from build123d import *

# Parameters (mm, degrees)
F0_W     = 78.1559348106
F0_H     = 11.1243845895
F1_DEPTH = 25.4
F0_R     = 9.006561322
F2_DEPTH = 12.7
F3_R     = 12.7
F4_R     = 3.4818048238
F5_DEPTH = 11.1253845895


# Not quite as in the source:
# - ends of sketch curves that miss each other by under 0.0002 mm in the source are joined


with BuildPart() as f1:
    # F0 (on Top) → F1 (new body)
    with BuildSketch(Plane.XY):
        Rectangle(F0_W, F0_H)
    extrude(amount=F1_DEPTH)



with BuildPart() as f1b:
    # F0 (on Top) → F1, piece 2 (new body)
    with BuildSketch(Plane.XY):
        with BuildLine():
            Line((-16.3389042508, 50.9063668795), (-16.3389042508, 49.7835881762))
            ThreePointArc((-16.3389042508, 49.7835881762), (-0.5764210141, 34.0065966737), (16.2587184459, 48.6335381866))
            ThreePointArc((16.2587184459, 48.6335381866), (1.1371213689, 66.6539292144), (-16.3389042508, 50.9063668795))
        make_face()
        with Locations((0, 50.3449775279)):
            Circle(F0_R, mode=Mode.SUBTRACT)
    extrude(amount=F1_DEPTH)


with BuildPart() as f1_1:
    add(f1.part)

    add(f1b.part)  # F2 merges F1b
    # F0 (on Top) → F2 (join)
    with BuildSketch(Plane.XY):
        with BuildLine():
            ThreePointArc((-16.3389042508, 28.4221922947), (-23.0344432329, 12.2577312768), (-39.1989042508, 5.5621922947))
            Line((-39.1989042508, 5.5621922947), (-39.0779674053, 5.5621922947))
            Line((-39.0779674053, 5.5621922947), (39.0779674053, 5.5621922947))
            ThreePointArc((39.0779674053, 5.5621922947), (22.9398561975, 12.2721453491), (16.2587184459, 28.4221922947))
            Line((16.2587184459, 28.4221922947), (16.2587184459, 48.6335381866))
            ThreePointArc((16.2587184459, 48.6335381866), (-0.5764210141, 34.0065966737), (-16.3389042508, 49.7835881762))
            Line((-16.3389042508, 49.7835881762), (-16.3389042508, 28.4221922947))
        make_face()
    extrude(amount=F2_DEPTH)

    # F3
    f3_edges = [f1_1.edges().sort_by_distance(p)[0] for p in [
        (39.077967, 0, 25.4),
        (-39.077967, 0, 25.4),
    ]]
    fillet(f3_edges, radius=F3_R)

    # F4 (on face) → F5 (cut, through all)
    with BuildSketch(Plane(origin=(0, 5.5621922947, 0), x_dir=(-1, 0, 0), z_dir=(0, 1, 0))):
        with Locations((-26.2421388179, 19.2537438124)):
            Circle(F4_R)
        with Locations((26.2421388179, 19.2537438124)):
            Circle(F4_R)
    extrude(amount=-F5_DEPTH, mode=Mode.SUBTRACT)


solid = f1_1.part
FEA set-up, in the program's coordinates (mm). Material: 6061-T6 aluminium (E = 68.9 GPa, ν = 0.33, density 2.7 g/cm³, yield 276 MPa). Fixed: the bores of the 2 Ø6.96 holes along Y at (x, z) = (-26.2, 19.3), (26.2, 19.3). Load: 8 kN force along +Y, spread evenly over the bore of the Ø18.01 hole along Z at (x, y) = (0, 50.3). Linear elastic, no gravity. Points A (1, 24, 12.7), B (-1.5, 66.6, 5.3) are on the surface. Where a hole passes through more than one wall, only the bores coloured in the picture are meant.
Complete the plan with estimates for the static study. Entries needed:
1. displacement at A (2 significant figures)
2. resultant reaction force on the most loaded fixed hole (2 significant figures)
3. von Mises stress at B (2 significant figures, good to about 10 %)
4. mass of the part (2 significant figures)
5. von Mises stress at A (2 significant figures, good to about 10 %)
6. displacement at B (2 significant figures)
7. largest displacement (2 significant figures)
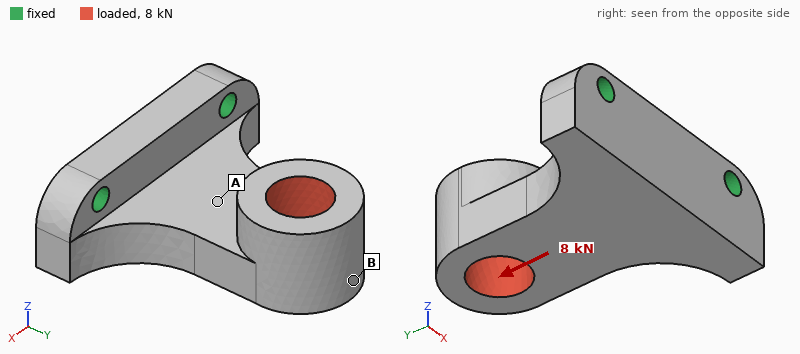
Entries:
0.035 mm
4.1 kN
14 MPa
140 g
62 MPa
0.17 mm
0.21 mm
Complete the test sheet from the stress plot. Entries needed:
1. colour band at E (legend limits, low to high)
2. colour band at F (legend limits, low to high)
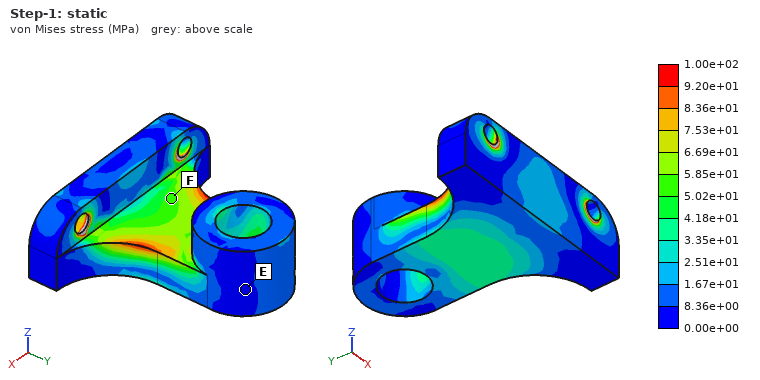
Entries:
0.00e+00 to 8.36e+00 MPa
5.02e+01 to 5.85e+01 MPa
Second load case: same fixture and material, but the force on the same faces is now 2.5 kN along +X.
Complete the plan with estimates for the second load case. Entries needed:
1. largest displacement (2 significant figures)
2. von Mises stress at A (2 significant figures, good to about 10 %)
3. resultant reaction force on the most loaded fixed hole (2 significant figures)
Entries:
0.10 mm
27 MPa
2.7 kN
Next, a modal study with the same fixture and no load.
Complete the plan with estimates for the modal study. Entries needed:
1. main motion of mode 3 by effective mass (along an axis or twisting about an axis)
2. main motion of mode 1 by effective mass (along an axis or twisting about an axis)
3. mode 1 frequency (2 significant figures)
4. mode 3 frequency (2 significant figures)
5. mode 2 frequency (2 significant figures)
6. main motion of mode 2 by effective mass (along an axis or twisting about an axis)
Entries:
along Y
along Z
1800 Hz
7000 Hz
4400 Hz
along X
